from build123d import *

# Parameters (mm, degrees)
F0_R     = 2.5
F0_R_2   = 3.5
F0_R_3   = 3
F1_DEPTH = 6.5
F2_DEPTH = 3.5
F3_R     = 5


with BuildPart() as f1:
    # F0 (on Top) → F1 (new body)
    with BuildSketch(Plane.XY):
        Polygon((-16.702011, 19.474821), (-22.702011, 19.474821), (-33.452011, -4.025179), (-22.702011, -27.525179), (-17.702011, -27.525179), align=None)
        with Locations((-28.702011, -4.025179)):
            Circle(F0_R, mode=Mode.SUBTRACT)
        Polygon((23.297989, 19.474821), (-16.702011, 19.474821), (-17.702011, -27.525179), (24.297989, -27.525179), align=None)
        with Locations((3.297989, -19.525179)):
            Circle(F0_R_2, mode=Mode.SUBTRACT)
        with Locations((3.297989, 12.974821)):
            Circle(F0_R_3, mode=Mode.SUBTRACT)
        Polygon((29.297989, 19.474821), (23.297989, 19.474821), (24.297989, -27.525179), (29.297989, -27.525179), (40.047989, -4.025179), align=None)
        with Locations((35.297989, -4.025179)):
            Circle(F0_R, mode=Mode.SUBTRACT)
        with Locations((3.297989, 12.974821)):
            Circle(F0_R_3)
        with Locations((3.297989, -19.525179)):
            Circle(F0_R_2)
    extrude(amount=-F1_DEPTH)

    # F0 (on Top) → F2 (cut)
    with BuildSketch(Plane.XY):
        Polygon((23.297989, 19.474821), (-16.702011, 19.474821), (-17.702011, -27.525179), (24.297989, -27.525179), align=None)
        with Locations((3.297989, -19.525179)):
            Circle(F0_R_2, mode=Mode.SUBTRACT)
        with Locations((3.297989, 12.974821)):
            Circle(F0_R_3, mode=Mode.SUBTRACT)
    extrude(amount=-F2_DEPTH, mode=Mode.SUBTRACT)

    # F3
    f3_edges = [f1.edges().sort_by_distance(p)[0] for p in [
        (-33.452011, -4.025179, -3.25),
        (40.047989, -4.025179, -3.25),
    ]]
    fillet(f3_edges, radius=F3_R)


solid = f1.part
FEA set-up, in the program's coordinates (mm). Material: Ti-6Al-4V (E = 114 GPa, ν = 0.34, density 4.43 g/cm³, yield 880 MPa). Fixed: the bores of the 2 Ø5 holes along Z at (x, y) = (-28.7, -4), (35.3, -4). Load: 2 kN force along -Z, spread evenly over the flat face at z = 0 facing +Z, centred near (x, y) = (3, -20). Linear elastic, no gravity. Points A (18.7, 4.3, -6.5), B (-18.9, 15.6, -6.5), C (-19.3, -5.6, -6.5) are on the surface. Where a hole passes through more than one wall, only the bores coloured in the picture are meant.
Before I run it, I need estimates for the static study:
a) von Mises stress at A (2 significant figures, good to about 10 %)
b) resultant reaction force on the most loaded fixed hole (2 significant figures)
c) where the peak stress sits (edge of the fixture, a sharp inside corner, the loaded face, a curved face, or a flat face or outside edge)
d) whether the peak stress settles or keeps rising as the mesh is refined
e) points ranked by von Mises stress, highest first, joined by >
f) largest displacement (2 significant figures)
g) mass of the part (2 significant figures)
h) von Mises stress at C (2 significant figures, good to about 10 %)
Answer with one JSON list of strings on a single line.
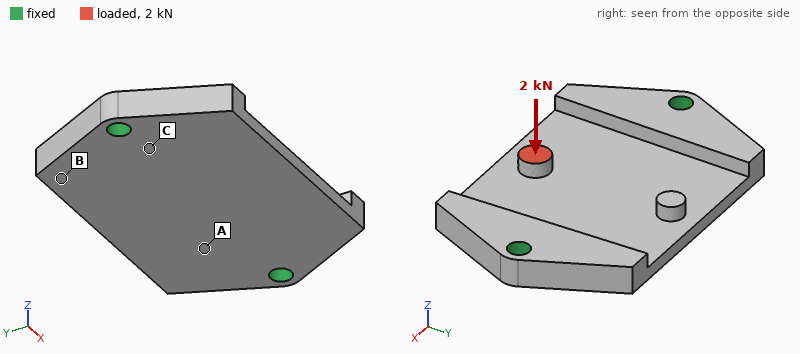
["64 MPa", "1.7 kN", "edge of the fixture", "keeps rising", "C > A > B", "0.34 mm", "55 g", "110 MPa"]
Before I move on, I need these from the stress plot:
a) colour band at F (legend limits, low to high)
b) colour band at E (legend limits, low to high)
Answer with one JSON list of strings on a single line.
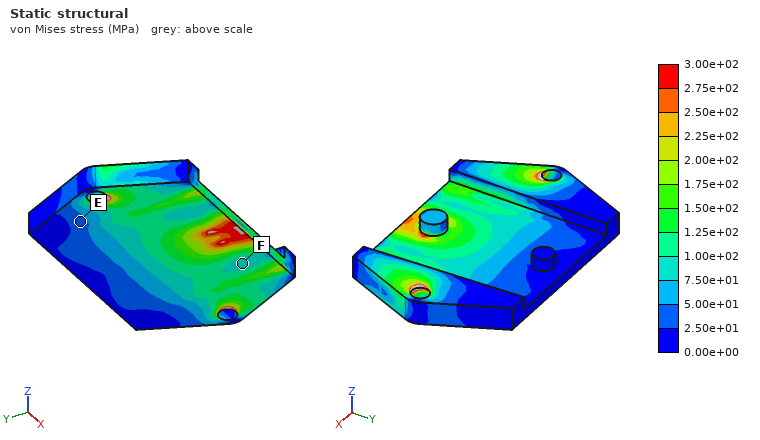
["7.50e+01 to 1.00e+02 MPa", "2.50e+01 to 5.00e+01 MPa"]
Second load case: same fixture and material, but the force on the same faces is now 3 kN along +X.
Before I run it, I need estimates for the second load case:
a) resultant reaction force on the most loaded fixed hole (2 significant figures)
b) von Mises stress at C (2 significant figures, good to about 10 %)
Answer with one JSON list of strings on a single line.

["1.7 kN", "53 MPa"]
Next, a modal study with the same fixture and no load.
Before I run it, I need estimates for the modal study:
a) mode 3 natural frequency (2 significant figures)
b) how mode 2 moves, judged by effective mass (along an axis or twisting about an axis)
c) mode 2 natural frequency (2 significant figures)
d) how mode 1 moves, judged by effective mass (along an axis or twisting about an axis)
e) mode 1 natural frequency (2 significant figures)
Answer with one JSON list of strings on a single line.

["9000 Hz", "along Z", "5400 Hz", "twisting about X", "5100 Hz"]
